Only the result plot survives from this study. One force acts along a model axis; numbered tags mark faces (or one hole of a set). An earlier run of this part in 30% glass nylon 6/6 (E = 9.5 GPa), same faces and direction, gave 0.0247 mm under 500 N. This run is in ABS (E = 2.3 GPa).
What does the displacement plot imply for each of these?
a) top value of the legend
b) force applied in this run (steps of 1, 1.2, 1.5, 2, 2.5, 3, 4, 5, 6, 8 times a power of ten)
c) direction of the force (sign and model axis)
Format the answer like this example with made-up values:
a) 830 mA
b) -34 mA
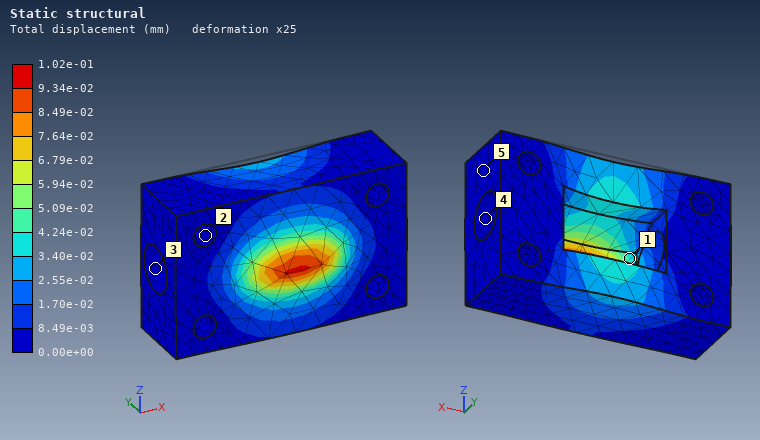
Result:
a) 1.02e-01 mm
b) 500 N
c) -Y
